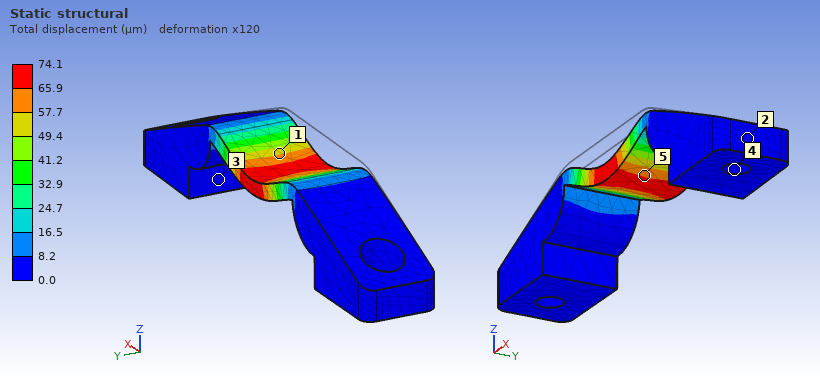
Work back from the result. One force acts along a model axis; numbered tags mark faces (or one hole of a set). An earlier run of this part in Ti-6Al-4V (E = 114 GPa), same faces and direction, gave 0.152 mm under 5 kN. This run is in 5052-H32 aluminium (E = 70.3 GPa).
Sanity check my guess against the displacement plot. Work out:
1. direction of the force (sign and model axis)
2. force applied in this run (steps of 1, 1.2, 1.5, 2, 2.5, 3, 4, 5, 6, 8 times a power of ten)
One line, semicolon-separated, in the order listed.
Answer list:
-Z; 1.5 kN
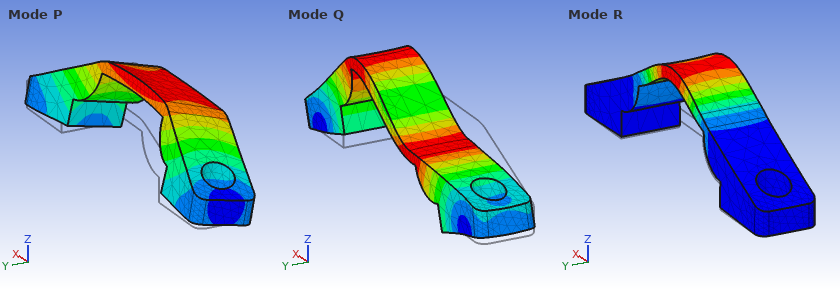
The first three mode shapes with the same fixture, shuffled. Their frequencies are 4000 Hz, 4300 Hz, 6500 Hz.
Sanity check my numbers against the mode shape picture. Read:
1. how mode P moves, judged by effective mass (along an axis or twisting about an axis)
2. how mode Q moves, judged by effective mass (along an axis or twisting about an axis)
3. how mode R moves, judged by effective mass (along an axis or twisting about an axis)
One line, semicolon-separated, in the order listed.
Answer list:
along Y; along X; along Z
